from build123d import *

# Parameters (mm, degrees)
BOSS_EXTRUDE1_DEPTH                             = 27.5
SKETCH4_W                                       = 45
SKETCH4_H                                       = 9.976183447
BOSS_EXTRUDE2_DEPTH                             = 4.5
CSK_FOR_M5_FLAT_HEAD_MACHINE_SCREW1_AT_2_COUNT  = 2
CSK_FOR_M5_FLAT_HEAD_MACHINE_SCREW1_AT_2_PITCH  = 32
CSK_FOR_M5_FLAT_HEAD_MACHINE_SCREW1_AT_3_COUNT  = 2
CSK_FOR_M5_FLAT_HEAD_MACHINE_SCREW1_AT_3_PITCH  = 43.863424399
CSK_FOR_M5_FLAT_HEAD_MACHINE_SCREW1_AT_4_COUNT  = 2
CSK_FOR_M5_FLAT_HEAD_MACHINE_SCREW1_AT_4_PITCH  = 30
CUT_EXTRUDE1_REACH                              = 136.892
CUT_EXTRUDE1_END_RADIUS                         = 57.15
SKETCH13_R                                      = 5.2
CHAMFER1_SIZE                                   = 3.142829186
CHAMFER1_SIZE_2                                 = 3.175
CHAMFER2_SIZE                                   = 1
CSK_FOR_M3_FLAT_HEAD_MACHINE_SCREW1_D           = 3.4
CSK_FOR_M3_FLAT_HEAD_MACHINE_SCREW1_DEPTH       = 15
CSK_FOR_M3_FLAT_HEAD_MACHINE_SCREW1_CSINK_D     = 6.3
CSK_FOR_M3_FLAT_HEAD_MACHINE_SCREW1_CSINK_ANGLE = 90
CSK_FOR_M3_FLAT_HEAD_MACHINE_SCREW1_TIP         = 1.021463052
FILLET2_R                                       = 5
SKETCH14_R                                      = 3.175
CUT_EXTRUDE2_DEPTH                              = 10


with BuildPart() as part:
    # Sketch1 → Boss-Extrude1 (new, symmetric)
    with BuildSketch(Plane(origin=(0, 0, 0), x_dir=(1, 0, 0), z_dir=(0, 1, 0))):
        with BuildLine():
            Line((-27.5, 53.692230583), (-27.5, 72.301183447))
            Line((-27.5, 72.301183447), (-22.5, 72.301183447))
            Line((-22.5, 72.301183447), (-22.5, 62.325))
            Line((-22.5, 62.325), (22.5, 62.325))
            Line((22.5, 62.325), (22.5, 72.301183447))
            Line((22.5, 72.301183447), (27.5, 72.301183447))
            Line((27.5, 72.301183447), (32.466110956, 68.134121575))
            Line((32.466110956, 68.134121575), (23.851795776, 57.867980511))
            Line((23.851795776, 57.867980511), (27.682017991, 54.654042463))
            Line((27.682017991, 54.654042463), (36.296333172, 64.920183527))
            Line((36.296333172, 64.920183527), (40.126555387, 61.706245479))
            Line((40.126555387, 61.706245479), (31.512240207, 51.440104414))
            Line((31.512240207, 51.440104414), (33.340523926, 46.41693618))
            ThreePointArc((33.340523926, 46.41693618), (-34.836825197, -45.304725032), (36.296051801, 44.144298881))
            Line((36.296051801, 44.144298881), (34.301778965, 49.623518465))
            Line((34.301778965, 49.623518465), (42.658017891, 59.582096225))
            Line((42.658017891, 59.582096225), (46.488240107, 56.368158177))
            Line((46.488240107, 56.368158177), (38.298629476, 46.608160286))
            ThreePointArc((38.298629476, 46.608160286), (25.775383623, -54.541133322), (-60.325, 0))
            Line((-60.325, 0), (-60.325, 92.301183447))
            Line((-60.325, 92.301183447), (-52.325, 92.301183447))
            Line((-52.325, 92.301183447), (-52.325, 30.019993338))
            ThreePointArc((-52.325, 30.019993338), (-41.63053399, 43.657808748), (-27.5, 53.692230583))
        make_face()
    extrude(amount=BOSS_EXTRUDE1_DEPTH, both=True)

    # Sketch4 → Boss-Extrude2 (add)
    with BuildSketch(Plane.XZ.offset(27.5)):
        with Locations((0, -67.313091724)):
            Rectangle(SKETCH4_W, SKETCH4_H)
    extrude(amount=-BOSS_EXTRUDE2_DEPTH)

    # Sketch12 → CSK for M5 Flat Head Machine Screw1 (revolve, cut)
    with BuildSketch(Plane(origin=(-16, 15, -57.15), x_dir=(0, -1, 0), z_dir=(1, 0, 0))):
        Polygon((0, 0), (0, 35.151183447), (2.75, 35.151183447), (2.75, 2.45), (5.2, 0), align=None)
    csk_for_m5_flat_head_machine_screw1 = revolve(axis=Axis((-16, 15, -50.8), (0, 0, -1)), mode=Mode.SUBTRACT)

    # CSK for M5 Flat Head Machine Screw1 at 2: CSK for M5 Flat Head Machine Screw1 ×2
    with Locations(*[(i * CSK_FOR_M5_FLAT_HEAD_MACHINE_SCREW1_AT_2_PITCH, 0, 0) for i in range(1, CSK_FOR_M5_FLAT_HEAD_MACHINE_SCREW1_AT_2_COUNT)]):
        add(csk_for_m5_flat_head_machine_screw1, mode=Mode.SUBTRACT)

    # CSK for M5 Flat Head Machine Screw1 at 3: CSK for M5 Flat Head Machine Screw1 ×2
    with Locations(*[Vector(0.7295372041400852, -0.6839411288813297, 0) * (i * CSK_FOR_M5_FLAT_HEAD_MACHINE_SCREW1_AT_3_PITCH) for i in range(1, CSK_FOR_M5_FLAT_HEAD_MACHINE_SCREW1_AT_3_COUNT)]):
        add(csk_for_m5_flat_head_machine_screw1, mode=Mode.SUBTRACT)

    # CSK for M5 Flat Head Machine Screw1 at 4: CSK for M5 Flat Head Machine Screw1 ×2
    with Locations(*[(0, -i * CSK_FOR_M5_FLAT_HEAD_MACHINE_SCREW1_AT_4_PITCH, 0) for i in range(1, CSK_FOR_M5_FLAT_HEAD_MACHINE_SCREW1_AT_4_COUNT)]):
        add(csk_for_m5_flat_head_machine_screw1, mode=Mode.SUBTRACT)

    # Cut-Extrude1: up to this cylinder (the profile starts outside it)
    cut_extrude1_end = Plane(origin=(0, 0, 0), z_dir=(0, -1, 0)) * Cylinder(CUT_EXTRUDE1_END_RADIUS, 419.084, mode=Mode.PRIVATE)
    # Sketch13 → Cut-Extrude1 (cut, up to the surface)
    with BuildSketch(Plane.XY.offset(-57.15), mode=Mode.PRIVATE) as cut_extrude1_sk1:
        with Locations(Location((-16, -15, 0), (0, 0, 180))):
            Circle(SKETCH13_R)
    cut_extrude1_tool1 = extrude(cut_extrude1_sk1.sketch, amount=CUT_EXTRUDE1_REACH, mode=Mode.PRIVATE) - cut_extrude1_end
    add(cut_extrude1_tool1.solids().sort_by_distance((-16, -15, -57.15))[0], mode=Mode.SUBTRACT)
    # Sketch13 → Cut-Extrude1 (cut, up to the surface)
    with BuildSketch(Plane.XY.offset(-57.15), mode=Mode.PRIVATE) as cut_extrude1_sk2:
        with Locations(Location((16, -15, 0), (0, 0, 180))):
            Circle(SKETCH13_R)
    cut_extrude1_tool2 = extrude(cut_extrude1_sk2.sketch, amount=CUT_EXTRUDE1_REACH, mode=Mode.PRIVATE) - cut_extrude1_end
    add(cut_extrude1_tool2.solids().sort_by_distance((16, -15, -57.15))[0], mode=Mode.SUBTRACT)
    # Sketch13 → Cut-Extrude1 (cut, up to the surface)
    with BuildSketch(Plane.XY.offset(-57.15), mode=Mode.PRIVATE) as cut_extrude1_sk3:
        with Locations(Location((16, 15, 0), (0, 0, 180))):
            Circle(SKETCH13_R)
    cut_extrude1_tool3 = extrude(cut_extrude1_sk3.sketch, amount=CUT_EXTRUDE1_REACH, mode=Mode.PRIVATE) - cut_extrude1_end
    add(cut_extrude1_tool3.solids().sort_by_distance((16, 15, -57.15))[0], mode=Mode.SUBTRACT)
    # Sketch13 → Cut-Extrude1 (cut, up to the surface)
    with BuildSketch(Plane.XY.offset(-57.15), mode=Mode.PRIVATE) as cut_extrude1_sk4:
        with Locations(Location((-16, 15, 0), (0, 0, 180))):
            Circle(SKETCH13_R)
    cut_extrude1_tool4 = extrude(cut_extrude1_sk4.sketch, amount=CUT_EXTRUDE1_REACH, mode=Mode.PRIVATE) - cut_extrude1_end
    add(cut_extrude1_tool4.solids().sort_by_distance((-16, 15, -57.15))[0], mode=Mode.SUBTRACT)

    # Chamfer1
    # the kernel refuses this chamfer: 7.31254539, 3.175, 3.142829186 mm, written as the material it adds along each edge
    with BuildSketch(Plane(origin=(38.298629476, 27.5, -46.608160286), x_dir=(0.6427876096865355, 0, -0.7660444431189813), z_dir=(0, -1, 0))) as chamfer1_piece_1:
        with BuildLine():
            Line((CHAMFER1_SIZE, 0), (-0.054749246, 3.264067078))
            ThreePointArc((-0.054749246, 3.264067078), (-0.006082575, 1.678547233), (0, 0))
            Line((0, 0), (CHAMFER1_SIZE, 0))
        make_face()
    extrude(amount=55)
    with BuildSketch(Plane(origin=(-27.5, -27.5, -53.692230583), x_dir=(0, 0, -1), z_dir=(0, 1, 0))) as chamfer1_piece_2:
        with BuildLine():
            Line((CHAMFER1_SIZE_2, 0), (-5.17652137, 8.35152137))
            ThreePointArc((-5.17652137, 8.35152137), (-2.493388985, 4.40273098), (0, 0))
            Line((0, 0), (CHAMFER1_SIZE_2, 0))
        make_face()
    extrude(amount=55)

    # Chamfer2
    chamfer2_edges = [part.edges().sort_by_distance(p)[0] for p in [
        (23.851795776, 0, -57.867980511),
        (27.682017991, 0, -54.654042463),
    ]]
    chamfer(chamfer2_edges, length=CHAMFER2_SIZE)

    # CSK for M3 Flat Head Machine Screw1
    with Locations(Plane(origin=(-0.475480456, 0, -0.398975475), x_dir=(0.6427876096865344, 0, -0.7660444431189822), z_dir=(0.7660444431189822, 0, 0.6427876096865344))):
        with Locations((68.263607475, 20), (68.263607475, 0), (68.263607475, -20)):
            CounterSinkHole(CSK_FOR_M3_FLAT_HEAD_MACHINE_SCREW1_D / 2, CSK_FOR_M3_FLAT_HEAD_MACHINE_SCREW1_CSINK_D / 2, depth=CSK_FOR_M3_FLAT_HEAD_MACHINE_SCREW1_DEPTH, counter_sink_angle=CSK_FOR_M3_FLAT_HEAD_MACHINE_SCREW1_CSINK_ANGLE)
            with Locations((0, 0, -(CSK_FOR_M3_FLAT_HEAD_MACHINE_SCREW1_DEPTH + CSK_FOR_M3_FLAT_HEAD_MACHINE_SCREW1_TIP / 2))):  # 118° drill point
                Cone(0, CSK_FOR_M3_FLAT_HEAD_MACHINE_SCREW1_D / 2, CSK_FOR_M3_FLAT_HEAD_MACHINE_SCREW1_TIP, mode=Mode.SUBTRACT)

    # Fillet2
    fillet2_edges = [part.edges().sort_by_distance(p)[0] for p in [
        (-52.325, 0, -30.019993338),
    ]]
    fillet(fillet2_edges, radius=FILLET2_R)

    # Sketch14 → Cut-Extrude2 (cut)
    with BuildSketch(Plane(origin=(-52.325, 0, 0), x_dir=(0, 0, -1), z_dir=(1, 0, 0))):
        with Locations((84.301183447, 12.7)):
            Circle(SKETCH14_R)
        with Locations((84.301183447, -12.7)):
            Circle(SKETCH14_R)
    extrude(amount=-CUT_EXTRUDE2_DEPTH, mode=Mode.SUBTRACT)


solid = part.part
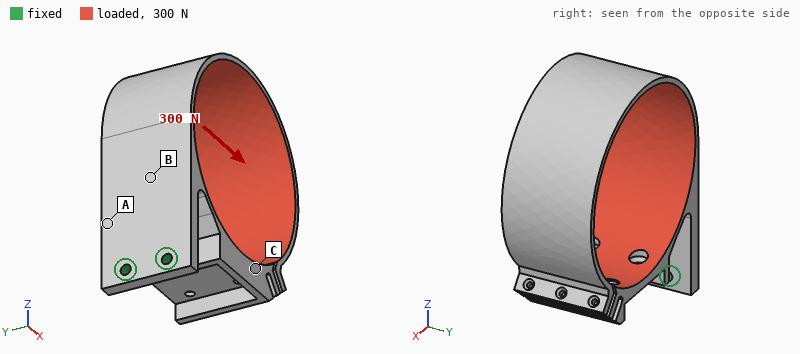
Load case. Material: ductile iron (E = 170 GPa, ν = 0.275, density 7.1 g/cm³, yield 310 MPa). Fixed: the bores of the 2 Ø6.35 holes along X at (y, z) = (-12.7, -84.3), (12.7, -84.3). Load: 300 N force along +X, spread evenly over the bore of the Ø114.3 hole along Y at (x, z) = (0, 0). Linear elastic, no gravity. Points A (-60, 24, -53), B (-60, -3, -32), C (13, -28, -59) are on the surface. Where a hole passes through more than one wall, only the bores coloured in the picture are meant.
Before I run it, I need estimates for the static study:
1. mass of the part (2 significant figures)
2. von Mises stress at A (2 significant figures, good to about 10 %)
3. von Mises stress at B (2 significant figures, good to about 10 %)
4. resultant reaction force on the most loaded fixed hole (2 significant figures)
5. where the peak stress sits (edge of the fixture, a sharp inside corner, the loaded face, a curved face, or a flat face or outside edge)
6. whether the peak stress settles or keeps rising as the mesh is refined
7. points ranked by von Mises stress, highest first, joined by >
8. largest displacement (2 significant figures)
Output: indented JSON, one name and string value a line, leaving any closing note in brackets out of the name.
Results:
{
  "mass of the part": "880 g",
  "von Mises stress at A": "28 MPa",
  "von Mises stress at B": "11 MPa",
  "resultant reaction force on the most loaded fixed hole": "150 N",
  "where the peak stress sits": "edge of the fixture",
  "whether the peak stress settles or keeps rising as the mesh is refined": "keeps rising",
  "points ranked by von Mises stress, highest first, joined by >": "A > B > C",
  "largest displacement": "2.0 mm"
}
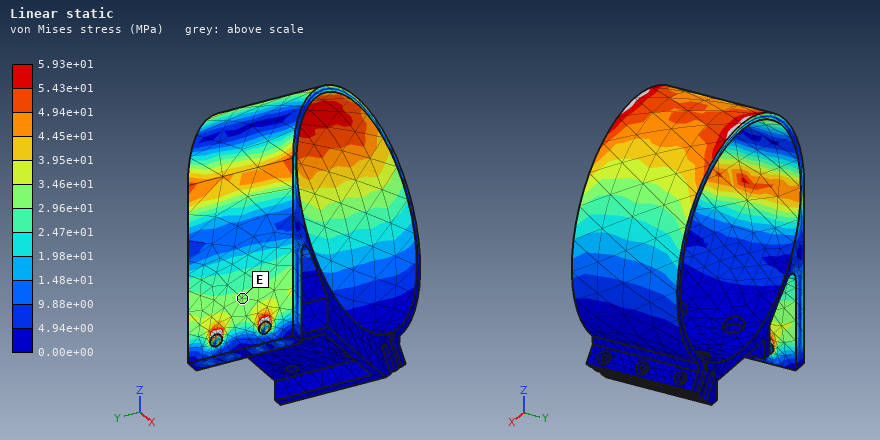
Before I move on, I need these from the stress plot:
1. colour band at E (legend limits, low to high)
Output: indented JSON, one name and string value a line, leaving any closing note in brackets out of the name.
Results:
{
  "colour band at E": "2.96e+01 to 3.46e+01 MPa"
}
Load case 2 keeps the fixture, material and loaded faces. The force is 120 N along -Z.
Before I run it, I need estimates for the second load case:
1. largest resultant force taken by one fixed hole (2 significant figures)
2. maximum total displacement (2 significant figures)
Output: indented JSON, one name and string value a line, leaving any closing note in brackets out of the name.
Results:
{
  "largest resultant force taken by one fixed hole": "60 N",
  "maximum total displacement": "2.3 mm"
}
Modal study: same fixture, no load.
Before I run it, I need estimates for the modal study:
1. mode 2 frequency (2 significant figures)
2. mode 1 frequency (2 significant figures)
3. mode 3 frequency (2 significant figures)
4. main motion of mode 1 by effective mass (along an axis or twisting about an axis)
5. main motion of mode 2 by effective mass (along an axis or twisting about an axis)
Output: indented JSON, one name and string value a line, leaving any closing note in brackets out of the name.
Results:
{
  "mode 2 frequency": "72 Hz",
  "mode 1 frequency": "53 Hz",
  "mode 3 frequency": "110 Hz",
  "main motion of mode 1 by effective mass": "along Z",
  "main motion of mode 2 by effective mass": "along Y"
}
